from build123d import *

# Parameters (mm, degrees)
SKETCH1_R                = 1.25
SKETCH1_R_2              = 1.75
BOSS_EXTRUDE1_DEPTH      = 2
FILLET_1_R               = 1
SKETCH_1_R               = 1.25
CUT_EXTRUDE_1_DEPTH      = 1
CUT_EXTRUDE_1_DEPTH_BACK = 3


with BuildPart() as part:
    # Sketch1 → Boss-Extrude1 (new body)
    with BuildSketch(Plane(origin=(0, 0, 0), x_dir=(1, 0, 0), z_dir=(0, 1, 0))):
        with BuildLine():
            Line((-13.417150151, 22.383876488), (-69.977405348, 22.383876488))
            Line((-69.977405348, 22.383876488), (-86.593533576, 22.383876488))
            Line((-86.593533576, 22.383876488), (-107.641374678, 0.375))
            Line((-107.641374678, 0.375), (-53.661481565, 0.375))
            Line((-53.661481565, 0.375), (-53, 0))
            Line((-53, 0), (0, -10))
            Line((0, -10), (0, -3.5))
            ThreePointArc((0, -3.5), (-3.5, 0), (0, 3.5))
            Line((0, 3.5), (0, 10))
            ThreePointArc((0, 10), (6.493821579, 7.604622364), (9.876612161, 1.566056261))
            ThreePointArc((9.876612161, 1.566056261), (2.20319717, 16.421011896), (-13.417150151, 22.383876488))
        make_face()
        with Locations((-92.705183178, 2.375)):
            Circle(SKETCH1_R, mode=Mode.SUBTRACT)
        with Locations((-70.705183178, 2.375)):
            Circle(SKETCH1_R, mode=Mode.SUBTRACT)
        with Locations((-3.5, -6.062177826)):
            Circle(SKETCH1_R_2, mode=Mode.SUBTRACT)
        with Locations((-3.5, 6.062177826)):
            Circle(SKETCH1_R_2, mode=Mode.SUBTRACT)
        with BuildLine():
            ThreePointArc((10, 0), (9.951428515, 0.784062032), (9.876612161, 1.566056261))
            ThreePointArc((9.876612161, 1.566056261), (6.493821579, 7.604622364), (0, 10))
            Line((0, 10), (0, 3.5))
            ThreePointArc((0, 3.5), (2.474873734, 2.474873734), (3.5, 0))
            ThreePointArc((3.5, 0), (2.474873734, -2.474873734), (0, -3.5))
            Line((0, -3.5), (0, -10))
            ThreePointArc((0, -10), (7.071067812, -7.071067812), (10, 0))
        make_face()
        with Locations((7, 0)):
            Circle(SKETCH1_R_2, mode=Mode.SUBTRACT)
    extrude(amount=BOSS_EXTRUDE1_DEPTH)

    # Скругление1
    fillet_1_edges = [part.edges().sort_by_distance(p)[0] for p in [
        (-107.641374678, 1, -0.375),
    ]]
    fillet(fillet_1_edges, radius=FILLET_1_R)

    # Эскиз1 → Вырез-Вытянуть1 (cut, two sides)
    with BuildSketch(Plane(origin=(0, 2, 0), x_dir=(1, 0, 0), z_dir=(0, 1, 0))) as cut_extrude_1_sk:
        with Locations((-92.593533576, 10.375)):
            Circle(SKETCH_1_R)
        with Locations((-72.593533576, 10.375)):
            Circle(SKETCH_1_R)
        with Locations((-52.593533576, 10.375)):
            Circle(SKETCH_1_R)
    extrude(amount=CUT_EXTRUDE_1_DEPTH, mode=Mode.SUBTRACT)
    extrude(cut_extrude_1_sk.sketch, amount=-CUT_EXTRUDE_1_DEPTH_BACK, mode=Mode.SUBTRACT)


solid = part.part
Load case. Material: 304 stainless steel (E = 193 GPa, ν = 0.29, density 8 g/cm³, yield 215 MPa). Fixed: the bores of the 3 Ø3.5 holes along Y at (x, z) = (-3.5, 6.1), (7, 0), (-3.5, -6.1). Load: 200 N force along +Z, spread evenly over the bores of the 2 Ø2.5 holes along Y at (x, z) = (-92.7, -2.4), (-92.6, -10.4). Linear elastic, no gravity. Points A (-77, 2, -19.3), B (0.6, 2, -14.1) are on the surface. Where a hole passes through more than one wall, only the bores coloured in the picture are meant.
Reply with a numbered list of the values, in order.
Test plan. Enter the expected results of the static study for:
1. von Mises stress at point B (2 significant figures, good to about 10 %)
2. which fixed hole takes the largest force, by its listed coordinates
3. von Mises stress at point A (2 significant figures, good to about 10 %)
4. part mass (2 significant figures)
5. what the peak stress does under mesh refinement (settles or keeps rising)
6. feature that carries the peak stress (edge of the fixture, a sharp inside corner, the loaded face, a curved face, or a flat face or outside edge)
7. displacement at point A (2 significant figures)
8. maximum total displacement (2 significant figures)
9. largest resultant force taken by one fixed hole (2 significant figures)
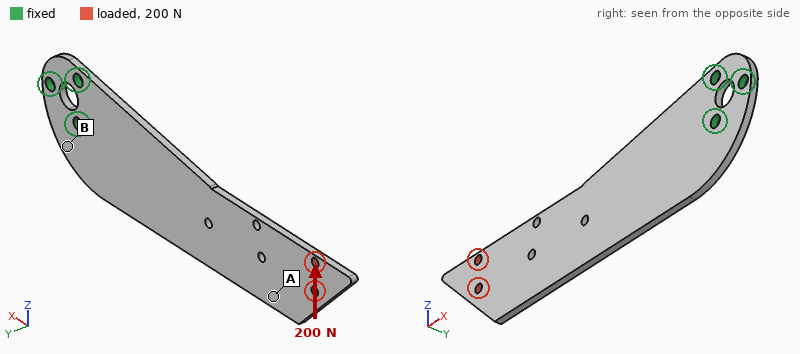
1. 37 MPa
2. (-3.5, 6.1)
3. 16 MPa
4. 40 g
5. keeps rising
6. edge of the fixture
7. 0.081 mm
8. 0.13 mm
9. 1.0 kN
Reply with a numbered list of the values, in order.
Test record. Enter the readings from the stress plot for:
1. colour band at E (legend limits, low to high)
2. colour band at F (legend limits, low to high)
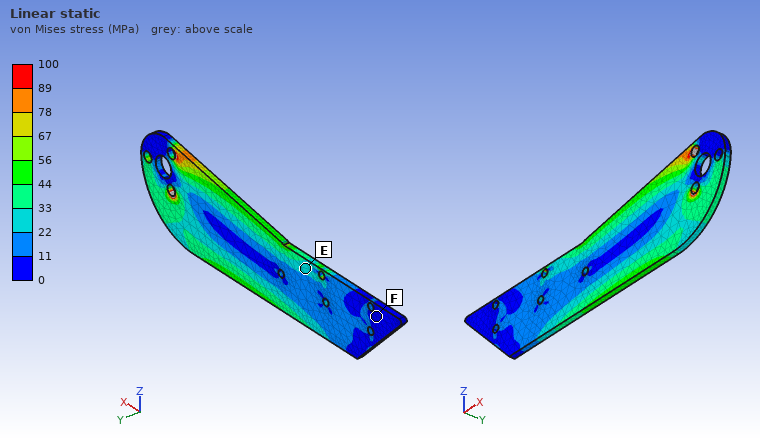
1. 22 to 33 MPa
2. 0 to 11 MPa
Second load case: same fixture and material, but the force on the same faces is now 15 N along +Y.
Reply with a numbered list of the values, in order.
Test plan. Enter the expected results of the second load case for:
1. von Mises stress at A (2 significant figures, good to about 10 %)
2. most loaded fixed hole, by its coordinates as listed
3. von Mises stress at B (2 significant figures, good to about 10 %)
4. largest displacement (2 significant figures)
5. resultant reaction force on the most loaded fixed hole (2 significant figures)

1. 17 MPa
2. (-3.5, -6.1)
3. 21 MPa
4. 1.3 mm
5. 29 N
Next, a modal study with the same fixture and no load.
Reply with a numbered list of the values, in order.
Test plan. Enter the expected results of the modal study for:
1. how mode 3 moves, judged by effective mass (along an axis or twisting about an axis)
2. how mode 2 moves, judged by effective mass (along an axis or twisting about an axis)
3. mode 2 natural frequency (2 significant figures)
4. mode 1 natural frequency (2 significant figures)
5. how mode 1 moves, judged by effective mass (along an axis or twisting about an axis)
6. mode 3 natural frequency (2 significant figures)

1. twisting about X
2. along Y
3. 1100 Hz
4. 200 Hz
5. along Y
6. 1700 Hz
